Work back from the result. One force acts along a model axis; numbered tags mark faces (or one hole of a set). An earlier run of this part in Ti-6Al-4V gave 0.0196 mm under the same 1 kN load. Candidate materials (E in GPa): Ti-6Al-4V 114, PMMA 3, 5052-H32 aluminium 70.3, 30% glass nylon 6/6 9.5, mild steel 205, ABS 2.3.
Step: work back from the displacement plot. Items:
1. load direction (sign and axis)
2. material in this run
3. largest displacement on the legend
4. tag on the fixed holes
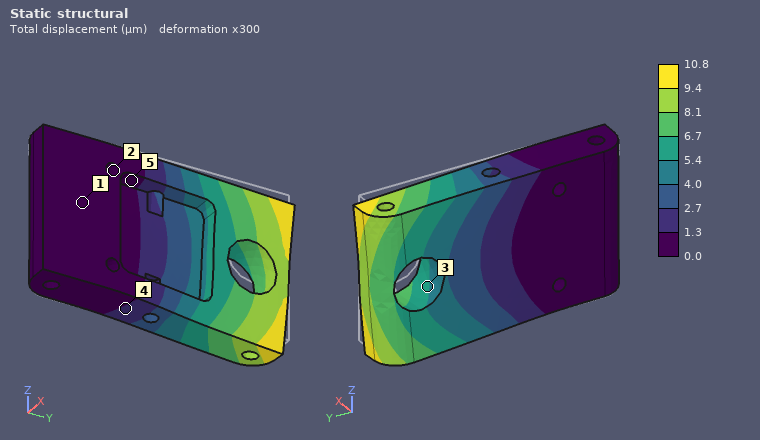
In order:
-Z
mild steel
10.8 µm
2
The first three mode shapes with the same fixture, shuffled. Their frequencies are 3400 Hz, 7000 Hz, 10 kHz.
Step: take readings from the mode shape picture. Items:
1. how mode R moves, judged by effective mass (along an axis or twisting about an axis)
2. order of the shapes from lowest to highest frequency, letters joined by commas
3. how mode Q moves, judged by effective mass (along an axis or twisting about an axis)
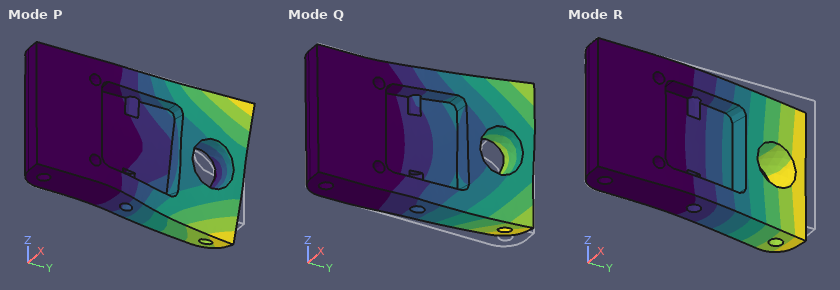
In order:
along X
R, P, Q
along Z
